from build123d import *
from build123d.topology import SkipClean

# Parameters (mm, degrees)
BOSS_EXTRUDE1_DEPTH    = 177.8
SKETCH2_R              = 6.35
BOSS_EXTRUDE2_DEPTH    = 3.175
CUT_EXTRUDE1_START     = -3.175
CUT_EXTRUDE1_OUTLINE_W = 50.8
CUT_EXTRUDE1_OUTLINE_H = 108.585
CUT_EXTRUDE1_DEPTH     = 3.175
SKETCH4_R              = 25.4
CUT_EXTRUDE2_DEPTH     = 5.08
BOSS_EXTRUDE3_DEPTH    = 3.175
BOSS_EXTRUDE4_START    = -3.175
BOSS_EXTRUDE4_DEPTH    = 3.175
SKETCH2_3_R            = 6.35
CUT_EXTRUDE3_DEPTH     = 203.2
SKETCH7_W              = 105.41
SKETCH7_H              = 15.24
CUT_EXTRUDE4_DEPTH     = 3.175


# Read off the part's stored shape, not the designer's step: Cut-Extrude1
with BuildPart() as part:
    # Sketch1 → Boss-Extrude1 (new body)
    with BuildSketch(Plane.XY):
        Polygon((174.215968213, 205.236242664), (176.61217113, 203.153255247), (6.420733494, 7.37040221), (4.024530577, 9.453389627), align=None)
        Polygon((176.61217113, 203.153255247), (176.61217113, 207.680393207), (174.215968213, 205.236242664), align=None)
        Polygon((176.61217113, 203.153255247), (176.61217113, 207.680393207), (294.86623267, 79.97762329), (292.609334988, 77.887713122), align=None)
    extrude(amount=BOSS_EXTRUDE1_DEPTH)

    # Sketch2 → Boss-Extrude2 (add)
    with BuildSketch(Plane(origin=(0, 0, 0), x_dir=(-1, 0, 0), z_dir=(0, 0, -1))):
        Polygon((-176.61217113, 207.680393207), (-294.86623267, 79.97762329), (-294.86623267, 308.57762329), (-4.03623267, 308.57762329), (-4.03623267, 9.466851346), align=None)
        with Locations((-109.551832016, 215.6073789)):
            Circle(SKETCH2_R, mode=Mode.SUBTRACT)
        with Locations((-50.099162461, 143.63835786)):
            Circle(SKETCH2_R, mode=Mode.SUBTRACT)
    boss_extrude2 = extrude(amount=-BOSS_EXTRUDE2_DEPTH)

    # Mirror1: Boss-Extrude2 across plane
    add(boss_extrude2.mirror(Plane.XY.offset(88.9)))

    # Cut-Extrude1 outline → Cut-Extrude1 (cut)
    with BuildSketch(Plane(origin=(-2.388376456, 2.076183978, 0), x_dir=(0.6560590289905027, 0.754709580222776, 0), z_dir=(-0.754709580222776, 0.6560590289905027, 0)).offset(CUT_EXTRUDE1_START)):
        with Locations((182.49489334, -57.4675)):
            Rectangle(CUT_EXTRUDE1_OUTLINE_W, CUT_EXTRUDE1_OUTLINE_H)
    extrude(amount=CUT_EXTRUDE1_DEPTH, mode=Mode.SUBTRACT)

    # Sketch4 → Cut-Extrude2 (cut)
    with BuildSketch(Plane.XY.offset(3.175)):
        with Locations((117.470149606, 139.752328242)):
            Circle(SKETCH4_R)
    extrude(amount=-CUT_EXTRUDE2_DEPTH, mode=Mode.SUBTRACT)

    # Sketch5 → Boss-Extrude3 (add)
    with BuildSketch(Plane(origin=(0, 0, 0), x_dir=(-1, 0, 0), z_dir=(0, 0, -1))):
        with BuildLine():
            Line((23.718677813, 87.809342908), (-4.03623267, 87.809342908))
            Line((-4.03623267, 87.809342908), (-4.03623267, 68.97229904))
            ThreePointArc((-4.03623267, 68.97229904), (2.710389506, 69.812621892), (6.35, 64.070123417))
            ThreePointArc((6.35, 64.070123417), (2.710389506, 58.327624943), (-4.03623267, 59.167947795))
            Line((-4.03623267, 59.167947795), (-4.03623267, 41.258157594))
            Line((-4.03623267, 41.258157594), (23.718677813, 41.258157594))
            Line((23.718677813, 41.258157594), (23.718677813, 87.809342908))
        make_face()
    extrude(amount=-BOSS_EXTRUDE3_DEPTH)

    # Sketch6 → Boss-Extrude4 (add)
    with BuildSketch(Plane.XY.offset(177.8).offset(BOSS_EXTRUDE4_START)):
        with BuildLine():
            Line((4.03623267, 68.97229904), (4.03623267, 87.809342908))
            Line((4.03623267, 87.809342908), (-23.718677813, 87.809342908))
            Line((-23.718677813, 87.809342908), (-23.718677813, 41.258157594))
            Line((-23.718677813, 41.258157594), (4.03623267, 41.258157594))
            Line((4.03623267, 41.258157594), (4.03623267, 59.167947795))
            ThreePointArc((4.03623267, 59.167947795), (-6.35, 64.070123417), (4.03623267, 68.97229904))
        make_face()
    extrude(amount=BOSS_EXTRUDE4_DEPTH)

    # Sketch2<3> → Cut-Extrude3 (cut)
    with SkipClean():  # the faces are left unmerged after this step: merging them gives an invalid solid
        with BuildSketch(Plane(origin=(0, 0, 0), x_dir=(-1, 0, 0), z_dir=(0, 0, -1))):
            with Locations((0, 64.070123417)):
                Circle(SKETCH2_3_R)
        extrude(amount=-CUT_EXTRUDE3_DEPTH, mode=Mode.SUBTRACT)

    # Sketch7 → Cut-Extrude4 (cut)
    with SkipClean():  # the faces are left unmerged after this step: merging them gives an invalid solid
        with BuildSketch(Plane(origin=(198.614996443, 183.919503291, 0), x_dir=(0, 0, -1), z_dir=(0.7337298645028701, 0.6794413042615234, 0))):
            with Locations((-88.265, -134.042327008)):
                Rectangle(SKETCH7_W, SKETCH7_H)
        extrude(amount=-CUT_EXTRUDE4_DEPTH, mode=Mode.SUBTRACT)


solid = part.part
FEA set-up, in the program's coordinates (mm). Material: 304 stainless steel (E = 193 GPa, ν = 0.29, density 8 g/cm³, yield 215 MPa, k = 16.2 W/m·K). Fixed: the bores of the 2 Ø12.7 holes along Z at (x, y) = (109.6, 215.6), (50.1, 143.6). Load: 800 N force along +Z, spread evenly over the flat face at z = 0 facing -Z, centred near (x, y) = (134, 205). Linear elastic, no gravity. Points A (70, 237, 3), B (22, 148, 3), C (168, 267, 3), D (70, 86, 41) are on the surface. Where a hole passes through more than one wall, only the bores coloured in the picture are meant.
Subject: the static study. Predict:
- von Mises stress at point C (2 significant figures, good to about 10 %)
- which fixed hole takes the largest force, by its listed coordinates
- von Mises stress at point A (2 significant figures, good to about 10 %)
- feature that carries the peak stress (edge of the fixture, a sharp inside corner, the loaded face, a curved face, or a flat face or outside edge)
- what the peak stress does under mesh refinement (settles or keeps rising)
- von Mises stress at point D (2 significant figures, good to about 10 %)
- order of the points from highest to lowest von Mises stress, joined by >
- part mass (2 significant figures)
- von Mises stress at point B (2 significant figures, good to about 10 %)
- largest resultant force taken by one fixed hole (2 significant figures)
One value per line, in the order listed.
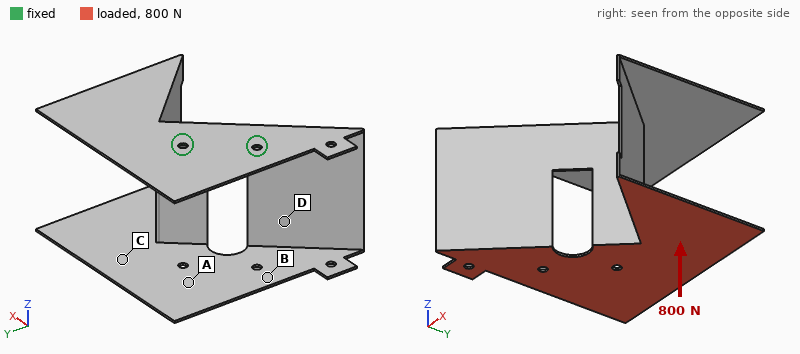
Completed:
53 MPa
(109.6, 215.6)
10 MPa
edge of the fixture
keeps rising
34 MPa
C > D > B > A
4.5 kg
21 MPa
760 N
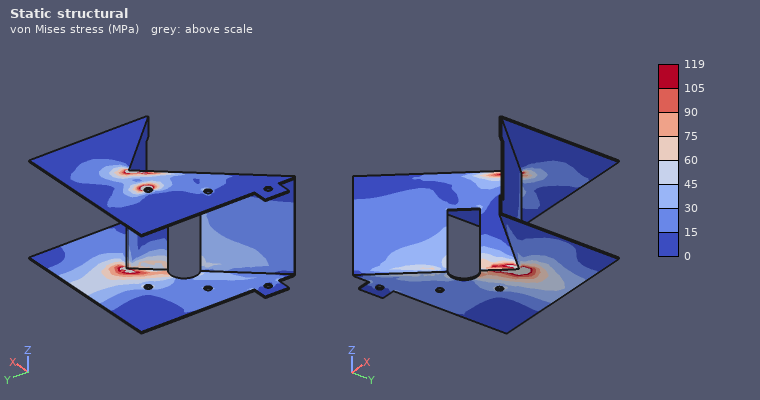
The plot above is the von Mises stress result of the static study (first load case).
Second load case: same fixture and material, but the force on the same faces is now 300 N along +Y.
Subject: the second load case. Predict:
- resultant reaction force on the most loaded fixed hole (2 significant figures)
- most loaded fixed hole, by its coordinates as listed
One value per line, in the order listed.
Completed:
460 N
(109.6, 215.6)
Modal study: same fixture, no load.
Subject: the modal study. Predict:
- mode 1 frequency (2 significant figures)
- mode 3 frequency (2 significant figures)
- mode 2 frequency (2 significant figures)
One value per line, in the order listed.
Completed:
23 Hz
67 Hz
46 Hz
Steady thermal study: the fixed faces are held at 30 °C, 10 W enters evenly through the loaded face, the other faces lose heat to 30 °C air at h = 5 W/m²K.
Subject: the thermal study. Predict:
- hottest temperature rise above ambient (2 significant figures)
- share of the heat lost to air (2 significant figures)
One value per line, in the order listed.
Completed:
28 K
99 %
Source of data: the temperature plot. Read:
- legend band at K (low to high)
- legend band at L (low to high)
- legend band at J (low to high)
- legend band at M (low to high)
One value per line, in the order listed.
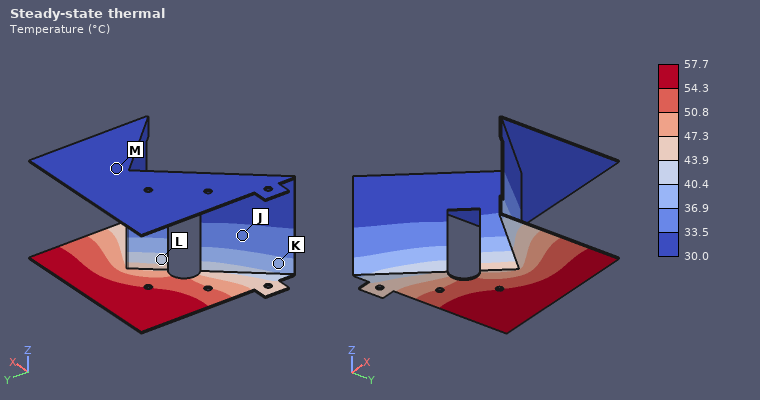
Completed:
36.9 to 40.4 °C
40.4 to 43.9 °C
33.5 to 36.9 °C
30.0 to 33.5 °C
